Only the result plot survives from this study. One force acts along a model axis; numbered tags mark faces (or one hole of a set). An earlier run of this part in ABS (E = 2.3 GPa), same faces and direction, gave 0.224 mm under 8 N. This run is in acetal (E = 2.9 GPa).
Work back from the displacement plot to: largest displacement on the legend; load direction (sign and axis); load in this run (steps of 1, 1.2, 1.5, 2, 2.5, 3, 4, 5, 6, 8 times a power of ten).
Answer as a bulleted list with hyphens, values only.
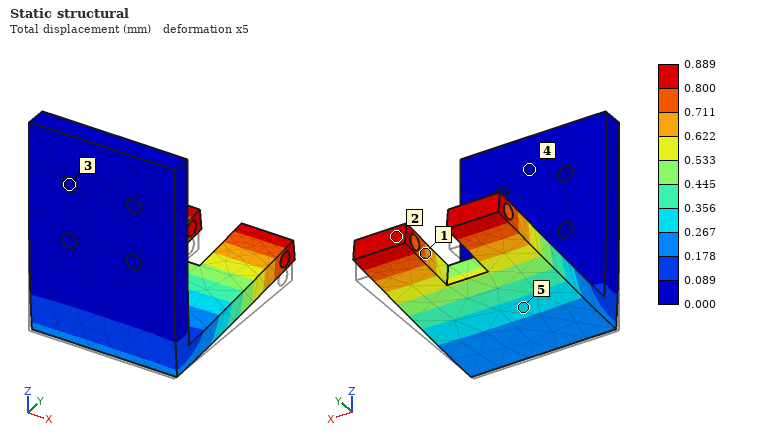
- 0.889 mm
- +Z
- 40 N
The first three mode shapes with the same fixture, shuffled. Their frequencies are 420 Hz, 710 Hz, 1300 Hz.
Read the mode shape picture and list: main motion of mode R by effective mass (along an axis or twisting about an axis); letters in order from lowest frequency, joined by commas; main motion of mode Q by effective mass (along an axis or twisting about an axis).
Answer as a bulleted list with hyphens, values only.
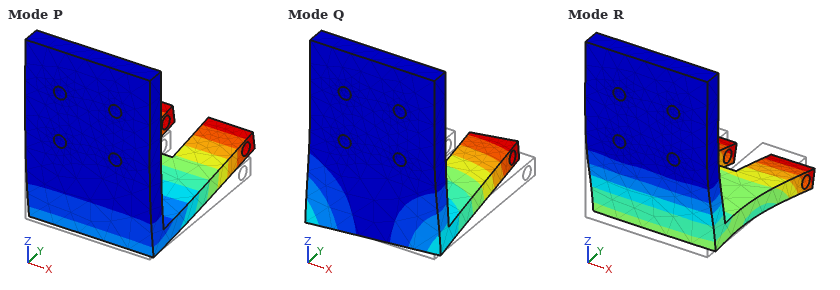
- along Y
- P, Q, R
- along X
